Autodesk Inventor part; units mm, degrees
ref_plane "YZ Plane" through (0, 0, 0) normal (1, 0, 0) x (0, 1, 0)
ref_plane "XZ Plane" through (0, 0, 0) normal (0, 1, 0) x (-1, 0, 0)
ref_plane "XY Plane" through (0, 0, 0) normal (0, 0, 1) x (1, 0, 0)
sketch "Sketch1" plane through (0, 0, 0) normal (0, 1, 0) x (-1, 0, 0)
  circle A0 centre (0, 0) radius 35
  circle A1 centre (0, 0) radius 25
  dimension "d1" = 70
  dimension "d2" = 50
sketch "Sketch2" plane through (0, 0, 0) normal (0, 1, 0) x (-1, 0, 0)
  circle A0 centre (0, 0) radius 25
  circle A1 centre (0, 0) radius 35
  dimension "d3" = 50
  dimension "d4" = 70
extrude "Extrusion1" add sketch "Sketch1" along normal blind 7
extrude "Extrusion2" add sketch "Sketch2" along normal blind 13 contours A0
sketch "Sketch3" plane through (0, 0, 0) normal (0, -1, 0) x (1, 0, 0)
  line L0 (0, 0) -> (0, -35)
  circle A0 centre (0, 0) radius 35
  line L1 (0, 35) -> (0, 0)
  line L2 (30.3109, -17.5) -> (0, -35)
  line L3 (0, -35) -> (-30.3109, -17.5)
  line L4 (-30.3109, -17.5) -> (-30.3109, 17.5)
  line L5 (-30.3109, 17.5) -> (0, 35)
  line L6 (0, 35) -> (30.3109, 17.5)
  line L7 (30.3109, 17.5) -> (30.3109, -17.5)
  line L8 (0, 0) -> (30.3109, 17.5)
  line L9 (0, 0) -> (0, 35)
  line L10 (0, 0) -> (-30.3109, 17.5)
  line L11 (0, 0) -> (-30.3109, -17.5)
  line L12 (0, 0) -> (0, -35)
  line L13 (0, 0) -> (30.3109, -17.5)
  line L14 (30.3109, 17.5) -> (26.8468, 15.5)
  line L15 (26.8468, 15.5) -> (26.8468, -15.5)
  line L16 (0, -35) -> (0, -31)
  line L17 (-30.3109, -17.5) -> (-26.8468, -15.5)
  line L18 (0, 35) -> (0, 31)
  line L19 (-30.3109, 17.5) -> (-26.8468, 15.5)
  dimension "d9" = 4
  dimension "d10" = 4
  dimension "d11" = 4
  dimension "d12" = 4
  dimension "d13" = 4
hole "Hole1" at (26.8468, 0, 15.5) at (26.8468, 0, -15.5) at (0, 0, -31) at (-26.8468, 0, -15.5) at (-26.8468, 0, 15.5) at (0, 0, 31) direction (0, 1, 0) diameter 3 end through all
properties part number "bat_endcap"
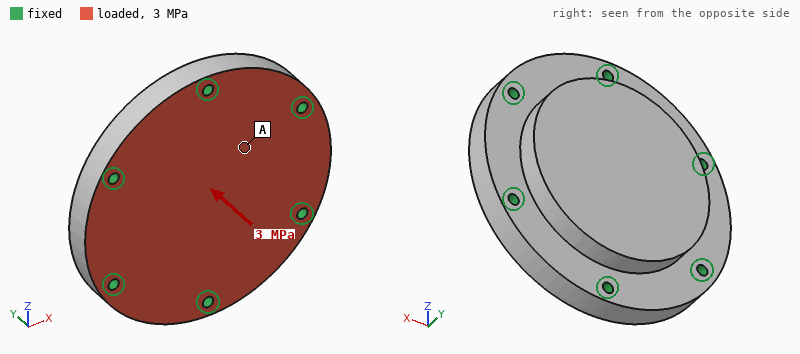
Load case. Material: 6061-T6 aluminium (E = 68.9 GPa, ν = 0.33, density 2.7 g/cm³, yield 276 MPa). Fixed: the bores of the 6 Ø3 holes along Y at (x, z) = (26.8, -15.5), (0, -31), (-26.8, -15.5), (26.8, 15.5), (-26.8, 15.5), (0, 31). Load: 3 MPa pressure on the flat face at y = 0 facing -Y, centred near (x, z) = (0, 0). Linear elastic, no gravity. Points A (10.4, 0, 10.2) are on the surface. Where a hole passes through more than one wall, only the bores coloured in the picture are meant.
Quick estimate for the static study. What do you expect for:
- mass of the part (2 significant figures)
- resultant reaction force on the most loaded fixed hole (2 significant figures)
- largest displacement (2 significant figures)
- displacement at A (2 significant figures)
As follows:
100 g
1.9 kN
15 µm
12 µm
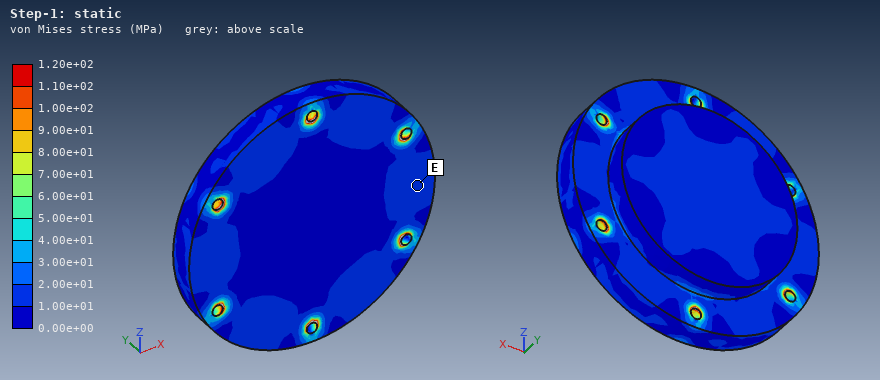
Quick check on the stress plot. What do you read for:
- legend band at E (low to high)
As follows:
1.00e+01 to 2.00e+01 MPa
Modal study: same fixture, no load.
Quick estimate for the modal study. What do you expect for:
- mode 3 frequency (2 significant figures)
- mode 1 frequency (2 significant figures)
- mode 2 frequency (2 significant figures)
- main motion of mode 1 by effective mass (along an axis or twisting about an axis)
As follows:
23 kHz
15 kHz
23 kHz
along Y
